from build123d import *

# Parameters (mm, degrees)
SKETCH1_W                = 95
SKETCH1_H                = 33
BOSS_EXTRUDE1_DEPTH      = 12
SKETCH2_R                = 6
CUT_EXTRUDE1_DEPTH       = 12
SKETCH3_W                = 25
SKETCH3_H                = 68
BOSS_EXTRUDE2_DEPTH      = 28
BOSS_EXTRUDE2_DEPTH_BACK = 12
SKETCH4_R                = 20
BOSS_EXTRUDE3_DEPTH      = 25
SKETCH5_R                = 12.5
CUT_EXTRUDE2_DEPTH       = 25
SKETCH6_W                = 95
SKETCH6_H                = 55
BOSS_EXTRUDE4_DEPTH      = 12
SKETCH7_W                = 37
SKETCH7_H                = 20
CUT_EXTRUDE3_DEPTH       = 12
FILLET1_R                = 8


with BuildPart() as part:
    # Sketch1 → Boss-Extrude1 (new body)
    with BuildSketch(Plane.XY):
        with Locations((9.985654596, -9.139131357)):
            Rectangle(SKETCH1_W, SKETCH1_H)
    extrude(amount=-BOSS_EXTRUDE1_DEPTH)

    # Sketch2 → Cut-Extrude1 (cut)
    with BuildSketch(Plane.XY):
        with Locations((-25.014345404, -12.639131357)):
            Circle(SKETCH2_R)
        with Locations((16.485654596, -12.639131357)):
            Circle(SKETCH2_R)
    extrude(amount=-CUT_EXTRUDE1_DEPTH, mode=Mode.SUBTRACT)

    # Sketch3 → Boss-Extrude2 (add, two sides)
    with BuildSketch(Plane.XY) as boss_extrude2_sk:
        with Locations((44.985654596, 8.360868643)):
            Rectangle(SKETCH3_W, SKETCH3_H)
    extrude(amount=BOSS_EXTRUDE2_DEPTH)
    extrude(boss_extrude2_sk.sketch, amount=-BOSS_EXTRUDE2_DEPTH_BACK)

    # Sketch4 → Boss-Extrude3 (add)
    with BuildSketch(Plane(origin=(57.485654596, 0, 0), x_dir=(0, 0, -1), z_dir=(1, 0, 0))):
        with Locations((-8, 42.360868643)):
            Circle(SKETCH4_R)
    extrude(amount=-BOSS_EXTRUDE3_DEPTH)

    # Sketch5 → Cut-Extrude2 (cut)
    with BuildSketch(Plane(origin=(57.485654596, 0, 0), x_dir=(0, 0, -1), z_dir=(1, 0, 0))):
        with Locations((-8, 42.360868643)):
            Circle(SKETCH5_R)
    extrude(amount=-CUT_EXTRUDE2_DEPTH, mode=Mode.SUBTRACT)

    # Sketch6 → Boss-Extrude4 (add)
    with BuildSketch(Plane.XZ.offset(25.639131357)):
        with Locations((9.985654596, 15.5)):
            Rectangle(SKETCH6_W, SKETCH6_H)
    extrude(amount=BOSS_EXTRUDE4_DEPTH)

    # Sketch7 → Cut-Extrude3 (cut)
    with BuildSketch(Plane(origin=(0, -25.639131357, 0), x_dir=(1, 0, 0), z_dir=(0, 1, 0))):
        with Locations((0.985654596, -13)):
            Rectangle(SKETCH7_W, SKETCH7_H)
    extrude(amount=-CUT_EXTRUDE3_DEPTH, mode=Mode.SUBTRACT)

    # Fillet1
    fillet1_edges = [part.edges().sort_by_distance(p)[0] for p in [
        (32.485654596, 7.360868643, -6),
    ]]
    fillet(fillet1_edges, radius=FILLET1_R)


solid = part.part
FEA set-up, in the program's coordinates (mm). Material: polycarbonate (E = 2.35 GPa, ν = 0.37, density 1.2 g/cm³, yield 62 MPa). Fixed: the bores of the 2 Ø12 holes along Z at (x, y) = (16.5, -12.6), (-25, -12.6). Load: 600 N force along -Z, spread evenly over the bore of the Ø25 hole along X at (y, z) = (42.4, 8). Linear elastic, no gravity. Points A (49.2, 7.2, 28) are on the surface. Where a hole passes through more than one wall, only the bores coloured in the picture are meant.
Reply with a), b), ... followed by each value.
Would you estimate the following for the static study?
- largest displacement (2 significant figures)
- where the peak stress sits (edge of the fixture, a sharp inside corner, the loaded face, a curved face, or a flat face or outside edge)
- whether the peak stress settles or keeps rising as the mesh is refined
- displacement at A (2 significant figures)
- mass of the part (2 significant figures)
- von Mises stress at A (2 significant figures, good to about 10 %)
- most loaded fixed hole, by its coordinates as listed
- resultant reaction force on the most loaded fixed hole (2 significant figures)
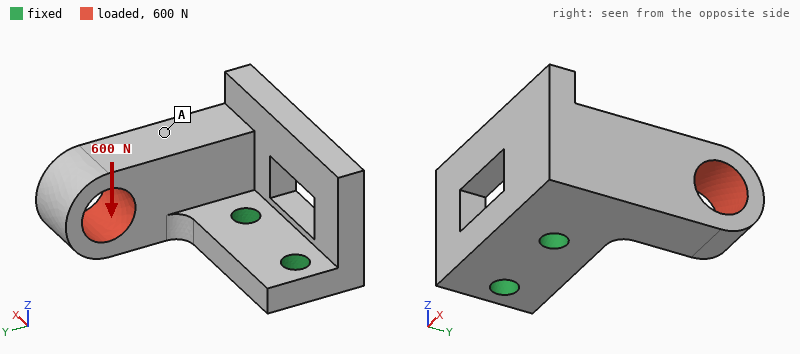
a) 1.8 mm
b) edge of the fixture
c) keeps rising
d) 0.78 mm
e) 180 g
f) 3.4 MPa
g) (16.5, -12.6)
h) 750 N
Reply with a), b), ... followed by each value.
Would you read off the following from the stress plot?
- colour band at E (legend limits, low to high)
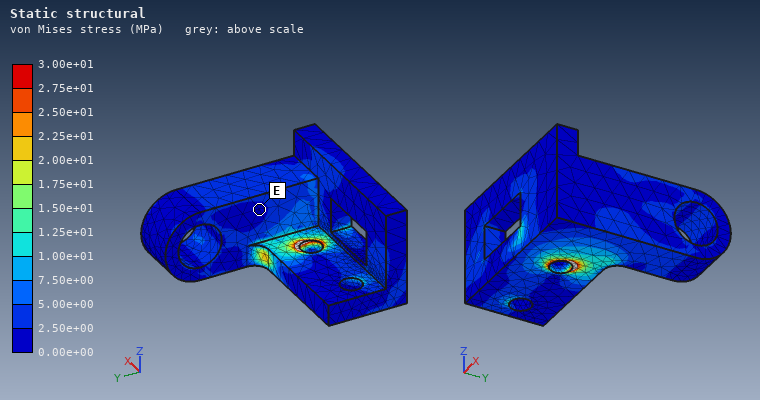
a) 0.00e+00 to 2.50e+00 MPa
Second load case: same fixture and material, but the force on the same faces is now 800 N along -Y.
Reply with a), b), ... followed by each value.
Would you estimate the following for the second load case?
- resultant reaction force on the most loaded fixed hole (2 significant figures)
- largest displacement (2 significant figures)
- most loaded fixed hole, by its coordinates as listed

a) 1.1 kN
b) 0.54 mm
c) (16.5, -12.6)
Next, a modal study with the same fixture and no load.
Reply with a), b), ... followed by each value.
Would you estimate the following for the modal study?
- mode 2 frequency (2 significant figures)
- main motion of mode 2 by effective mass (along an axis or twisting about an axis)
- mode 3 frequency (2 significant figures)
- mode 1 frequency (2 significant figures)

a) 670 Hz
b) along X
c) 970 Hz
d) 500 Hz
